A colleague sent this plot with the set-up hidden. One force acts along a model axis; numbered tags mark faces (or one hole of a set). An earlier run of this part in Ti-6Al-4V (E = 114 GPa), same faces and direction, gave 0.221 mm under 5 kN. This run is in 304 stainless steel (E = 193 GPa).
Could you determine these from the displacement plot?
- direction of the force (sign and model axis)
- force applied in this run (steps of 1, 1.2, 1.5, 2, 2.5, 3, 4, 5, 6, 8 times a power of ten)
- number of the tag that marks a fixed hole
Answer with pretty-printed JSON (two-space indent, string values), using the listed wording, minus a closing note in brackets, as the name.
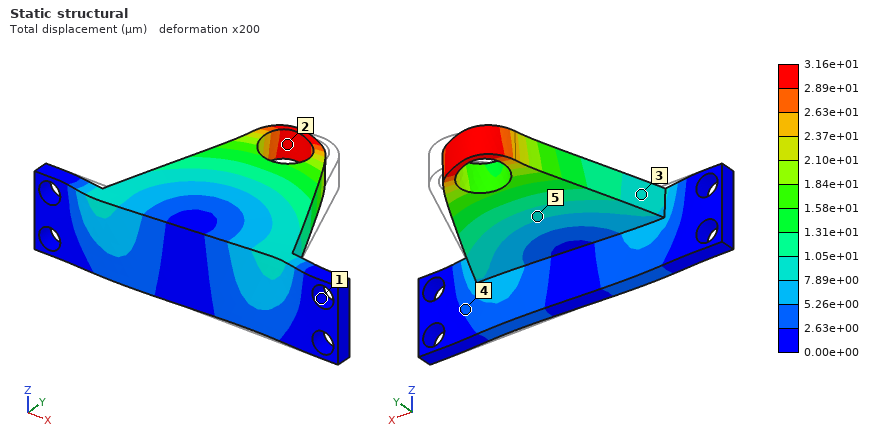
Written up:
{
  "direction of the force": "-X",
  "force applied in this run": "1.2 kN",
  "number of the tag that marks a fixed hole": "1"
}
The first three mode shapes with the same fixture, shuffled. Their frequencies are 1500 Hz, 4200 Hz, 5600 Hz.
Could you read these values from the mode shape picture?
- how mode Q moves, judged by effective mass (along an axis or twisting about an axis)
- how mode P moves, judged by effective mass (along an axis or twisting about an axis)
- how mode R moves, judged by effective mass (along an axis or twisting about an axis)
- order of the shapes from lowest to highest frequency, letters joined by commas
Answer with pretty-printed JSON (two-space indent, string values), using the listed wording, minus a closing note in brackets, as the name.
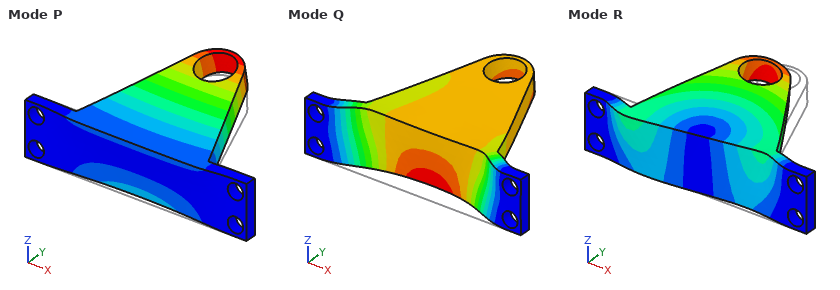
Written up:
{
  "how mode Q moves, judged by effective mass": "along Y",
  "how mode P moves, judged by effective mass": "along Z",
  "how mode R moves, judged by effective mass": "along X",
  "order of the shapes from lowest to highest frequency, letters joined by commas": "P, Q, R"
}
